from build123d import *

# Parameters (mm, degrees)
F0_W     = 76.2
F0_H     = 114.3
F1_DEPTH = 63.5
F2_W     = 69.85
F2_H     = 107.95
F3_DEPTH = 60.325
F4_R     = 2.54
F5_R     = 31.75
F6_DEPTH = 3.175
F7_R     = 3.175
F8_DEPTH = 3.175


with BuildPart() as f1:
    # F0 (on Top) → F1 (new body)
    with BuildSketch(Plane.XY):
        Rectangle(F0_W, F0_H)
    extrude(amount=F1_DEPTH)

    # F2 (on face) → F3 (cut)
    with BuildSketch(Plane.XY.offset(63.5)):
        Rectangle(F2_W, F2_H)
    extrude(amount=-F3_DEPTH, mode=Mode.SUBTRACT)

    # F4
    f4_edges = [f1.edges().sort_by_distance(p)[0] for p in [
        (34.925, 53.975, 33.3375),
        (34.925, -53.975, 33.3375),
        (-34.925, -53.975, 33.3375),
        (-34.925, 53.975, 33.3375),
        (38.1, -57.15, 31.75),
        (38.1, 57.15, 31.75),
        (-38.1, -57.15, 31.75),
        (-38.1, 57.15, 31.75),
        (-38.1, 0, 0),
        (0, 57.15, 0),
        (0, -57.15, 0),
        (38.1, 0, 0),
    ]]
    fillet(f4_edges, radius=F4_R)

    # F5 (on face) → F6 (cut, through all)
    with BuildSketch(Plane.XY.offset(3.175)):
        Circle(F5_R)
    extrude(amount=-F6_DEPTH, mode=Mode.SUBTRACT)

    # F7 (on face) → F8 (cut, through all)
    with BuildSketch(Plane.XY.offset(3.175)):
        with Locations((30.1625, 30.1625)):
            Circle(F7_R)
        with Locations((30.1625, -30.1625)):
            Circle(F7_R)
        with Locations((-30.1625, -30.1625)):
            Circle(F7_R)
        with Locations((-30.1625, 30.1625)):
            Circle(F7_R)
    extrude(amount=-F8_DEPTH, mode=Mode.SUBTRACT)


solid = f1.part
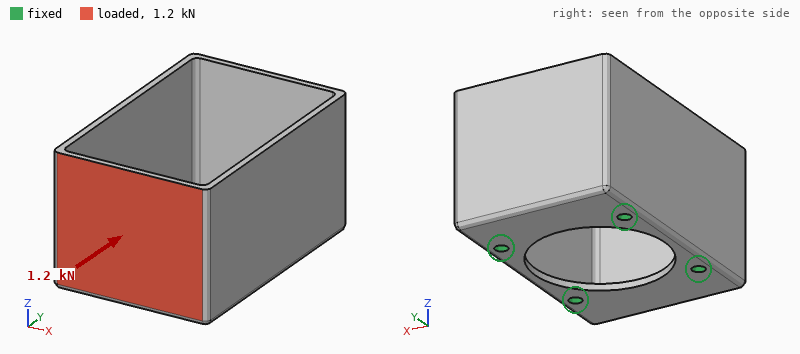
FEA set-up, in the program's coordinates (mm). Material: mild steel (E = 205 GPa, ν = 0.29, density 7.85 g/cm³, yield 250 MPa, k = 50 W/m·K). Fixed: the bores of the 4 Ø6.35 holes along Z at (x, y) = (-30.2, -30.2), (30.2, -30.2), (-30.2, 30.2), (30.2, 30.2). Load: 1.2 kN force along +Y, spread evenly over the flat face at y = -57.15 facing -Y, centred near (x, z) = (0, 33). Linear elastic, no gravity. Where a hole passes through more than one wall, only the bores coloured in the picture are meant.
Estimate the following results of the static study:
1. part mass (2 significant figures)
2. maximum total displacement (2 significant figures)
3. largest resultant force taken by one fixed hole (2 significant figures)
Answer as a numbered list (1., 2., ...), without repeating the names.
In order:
1. 680 g
2. 81 µm
3. 540 N
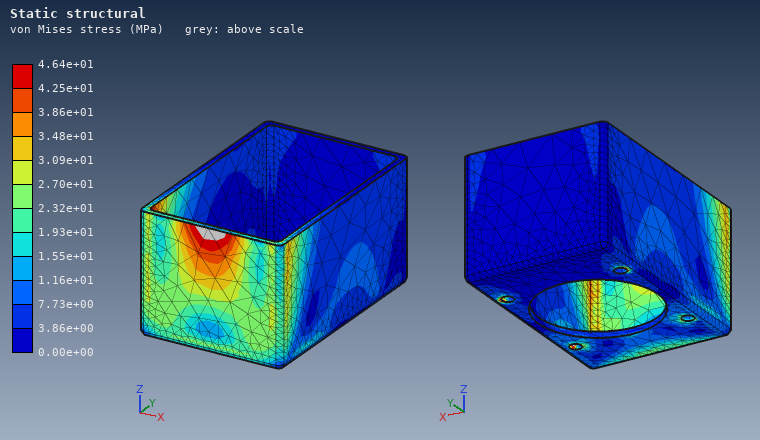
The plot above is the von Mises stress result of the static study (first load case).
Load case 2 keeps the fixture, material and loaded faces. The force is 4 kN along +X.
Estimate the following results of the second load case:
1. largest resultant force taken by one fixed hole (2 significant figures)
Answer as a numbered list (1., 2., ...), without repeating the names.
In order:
1. 3.6 kN
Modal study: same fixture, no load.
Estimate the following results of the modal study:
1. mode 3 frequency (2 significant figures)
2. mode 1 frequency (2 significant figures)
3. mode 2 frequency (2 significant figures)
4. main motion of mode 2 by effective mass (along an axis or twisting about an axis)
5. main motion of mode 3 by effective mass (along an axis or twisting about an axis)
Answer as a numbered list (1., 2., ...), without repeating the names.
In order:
1. 2300 Hz
2. 1300 Hz
3. 1400 Hz
4. along X
5. along Y
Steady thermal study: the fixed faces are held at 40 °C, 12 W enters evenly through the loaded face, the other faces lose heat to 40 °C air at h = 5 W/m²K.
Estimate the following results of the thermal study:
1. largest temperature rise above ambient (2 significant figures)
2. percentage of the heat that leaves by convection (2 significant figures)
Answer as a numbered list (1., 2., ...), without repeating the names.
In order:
1. 28 K
2. 15 %
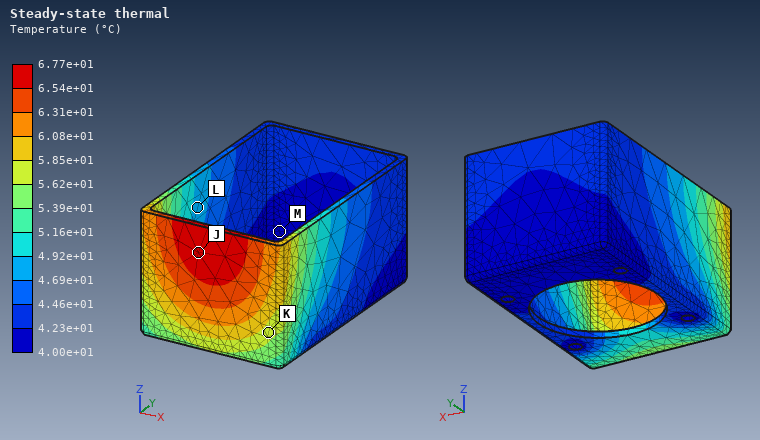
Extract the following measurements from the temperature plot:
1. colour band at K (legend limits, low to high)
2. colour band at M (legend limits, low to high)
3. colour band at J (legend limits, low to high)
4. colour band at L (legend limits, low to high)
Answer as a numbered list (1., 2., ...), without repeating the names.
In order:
1. 5.62e+01 to 5.85e+01 °C
2. 4.00e+01 to 4.23e+01 °C
3. 6.54e+01 to 6.77e+01 °C
4. 4.69e+01 to 4.92e+01 °C
